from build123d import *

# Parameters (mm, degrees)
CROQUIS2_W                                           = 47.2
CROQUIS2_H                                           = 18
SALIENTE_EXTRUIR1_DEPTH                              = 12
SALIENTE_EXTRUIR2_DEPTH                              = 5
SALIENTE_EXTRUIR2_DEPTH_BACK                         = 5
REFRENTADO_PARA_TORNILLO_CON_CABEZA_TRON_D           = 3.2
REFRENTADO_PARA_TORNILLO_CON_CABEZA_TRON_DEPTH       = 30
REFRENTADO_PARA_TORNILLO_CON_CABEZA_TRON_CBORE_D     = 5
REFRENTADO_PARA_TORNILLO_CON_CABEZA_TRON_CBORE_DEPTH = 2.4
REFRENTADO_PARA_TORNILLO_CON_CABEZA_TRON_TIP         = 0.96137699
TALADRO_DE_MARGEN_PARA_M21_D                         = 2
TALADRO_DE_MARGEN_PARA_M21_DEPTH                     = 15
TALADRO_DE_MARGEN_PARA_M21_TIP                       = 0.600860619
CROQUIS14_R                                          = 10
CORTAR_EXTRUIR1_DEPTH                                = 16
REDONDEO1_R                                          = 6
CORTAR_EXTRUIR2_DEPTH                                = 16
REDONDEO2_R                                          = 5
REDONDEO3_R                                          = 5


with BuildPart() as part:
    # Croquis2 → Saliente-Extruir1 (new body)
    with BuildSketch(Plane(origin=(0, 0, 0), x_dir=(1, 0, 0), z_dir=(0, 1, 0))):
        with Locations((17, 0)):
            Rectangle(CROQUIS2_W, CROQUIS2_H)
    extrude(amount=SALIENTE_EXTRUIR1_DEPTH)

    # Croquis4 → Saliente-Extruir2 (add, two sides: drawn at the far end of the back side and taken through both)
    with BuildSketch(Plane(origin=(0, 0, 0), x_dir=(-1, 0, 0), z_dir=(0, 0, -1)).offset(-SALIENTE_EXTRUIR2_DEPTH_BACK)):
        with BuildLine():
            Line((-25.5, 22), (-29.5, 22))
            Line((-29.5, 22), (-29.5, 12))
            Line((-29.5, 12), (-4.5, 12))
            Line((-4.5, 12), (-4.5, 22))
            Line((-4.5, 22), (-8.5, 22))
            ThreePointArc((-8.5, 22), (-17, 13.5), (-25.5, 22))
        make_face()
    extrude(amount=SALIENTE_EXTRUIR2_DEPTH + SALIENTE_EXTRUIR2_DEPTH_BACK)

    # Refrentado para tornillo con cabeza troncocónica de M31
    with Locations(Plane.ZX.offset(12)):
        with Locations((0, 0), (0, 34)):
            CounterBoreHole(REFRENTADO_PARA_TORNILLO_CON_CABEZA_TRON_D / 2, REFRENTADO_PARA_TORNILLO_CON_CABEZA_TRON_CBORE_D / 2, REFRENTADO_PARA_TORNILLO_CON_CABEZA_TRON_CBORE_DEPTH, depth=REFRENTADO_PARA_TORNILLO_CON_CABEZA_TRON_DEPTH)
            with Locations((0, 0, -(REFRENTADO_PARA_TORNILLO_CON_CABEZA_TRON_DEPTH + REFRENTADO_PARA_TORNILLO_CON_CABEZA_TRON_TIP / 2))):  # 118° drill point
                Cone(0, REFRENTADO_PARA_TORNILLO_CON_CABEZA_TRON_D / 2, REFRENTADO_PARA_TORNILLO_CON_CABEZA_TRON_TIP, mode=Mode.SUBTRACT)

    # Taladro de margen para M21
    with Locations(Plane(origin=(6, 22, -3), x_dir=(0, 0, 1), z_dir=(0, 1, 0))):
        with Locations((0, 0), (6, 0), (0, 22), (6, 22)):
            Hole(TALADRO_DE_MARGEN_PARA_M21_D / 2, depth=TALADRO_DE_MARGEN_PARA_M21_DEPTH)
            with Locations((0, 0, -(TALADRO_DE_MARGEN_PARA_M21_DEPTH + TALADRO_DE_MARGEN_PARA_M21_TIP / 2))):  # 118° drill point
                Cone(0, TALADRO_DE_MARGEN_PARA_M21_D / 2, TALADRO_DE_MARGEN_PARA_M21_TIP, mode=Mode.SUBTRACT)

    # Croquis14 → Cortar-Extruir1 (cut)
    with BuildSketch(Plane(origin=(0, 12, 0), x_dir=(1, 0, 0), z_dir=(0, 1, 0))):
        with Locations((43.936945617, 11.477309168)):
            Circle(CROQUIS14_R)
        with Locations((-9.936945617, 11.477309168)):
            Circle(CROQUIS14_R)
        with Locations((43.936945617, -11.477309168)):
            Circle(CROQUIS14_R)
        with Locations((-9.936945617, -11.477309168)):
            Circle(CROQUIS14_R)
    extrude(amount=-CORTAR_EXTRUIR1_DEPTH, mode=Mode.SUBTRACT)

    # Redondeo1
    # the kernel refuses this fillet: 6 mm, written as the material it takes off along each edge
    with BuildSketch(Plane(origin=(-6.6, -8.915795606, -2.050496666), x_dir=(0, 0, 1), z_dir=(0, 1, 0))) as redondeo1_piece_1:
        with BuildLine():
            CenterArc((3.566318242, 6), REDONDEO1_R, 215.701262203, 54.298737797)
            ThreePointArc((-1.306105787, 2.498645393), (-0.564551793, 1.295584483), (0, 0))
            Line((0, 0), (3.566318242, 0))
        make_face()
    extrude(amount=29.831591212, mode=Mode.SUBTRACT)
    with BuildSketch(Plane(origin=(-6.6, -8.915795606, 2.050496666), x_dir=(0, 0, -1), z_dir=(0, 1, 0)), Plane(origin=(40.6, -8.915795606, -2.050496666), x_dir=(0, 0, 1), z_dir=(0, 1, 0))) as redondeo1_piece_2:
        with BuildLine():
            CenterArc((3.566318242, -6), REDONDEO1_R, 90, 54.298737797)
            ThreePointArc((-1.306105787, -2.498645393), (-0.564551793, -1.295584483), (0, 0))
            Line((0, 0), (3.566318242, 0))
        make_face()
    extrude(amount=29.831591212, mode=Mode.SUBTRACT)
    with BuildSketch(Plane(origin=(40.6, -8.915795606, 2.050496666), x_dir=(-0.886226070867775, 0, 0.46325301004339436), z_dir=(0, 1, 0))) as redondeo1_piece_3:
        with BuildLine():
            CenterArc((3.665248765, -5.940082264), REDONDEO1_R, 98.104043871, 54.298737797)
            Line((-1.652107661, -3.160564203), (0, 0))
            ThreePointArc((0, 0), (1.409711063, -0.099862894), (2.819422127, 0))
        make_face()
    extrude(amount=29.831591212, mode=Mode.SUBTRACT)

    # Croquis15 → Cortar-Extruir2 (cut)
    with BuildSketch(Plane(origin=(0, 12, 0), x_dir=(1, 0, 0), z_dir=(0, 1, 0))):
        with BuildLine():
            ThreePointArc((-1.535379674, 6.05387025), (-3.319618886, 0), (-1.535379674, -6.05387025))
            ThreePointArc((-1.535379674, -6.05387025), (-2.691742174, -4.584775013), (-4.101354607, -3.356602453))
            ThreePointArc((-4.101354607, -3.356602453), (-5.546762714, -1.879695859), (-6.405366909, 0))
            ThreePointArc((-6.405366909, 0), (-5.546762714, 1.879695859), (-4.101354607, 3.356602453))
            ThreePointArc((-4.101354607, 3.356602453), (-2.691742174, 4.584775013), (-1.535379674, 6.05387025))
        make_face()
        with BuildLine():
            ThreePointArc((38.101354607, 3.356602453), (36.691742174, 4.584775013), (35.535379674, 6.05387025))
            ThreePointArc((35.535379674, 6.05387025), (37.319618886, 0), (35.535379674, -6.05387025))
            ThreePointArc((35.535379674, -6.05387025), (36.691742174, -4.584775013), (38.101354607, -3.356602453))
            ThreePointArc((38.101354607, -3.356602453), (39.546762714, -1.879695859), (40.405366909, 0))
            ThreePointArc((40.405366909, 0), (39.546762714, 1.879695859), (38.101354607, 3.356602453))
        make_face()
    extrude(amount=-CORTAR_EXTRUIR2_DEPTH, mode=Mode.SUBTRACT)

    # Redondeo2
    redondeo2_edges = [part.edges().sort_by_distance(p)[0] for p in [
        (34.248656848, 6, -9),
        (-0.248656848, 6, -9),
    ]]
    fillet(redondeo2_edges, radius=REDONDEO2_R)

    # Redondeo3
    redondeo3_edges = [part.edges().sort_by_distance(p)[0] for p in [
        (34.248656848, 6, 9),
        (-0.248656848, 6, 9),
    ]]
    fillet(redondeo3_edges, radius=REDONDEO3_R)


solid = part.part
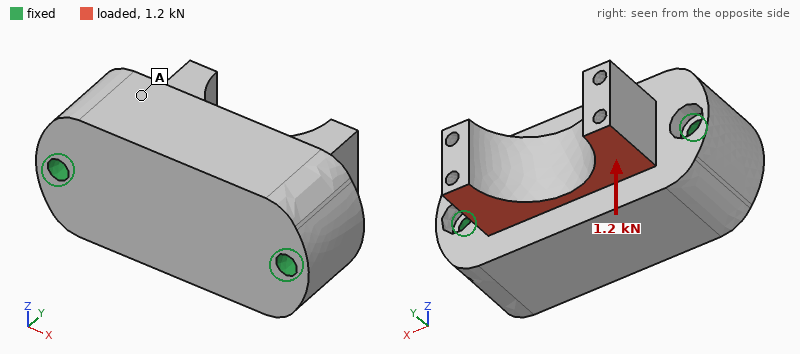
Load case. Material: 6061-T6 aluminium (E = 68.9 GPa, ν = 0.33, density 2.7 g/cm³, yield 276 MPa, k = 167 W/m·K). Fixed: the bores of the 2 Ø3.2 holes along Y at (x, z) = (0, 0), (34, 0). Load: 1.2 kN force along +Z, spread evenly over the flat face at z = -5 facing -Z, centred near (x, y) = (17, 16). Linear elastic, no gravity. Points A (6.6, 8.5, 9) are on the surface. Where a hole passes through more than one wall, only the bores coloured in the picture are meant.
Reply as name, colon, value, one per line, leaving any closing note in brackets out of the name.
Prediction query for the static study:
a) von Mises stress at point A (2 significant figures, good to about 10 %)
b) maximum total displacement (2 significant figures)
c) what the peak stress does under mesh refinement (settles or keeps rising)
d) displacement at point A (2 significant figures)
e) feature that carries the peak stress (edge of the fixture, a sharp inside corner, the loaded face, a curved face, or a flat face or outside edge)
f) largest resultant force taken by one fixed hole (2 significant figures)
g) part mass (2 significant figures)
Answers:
von Mises stress at point A: 12 MPa
maximum total displacement: 18 µm
what the peak stress does under mesh refinement: keeps rising
displacement at point A: 5.7 µm
feature that carries the peak stress: edge of the fixture
largest resultant force taken by one fixed hole: 600 N
part mass: 25 g
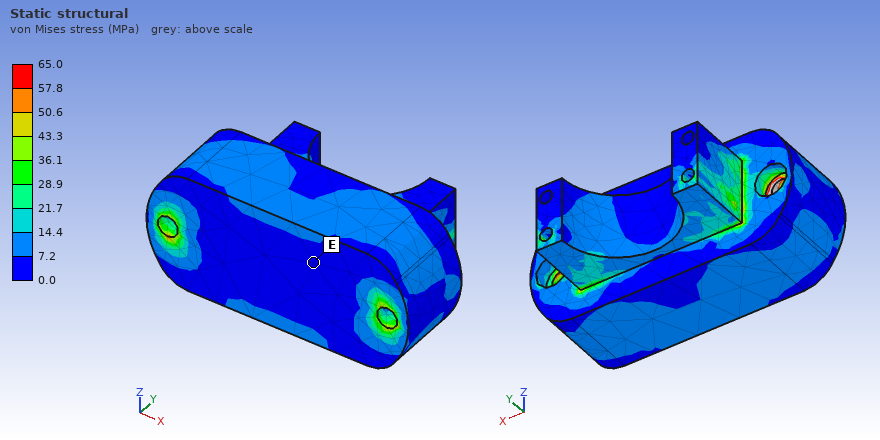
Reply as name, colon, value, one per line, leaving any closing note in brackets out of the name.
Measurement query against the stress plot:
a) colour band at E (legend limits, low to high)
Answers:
colour band at E: 0.0 to 7.2 MPa
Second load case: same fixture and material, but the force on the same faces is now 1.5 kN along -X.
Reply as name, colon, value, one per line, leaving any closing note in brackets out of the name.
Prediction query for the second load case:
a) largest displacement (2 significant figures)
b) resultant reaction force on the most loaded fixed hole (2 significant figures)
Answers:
largest displacement: 16 µm
resultant reaction force on the most loaded fixed hole: 910 N
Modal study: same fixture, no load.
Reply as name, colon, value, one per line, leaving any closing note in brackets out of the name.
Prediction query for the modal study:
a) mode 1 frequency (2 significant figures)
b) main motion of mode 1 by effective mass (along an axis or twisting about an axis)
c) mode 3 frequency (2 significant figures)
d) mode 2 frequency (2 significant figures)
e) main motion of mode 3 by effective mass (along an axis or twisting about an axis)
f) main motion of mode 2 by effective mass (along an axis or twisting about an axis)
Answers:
mode 1 frequency: 21 kHz
main motion of mode 1 by effective mass: along Z
mode 3 frequency: 29 kHz
mode 2 frequency: 25 kHz
main motion of mode 3 by effective mass: along Z
main motion of mode 2 by effective mass: along Y
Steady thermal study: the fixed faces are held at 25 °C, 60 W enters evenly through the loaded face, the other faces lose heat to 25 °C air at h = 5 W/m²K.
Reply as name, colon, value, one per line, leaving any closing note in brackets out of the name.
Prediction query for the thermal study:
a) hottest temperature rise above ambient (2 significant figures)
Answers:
hottest temperature rise above ambient: 37 K
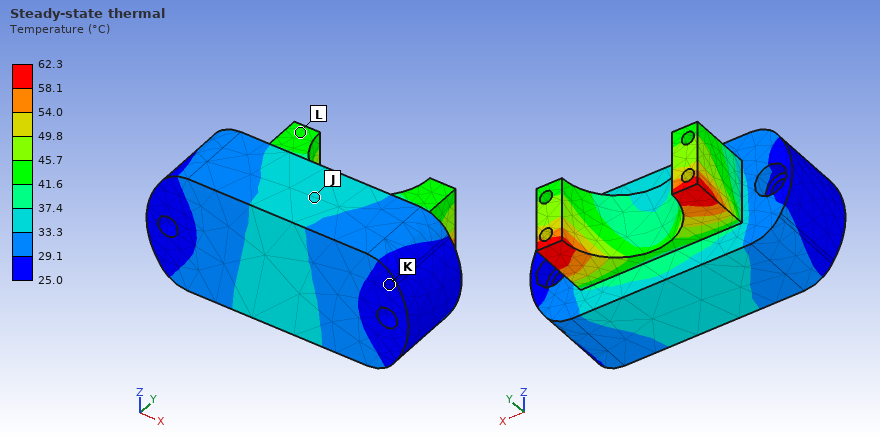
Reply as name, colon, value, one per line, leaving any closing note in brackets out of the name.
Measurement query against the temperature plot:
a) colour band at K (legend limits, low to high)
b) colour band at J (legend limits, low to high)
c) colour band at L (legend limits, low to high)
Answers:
colour band at K: 25.0 to 29.1 °C
colour band at J: 33.3 to 37.4 °C
colour band at L: 41.6 to 45.7 °C
